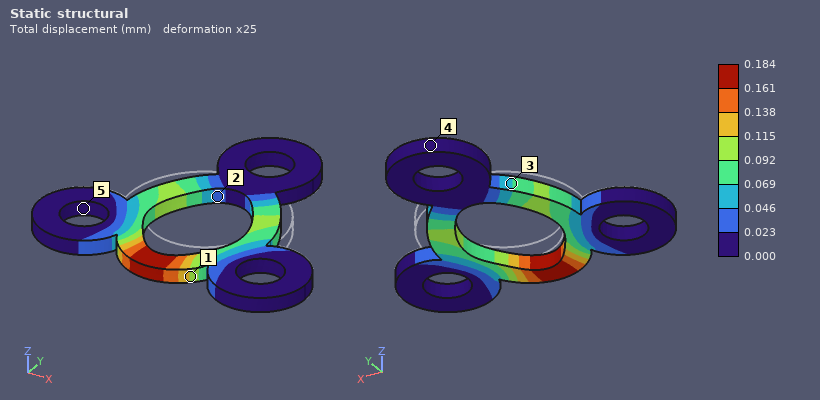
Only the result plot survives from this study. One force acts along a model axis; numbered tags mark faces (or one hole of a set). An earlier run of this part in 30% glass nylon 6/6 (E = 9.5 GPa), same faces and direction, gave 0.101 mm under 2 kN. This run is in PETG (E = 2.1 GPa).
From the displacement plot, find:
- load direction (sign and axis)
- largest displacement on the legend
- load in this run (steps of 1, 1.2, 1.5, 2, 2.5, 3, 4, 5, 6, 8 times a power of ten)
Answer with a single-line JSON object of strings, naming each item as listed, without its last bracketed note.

{"load direction": "-Y", "largest displacement on the legend": "0.184 mm", "load in this run": "800 N"}
